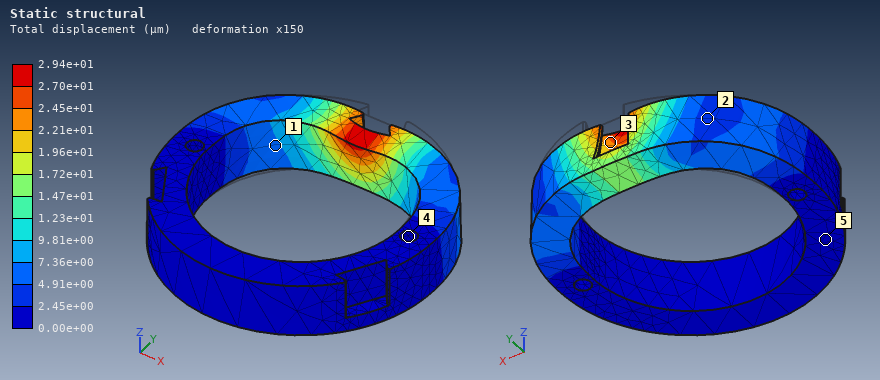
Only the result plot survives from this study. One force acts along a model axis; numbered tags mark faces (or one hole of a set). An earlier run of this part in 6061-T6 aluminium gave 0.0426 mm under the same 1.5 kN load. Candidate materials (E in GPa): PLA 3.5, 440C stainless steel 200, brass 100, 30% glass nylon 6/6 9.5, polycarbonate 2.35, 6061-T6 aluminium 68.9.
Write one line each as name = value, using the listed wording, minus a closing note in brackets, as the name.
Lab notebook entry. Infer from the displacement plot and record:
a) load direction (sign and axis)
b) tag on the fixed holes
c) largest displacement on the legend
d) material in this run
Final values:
load direction = -Y
tag on the fixed holes = 4
largest displacement on the legend = 2.94e+01 µm
material in this run = brass
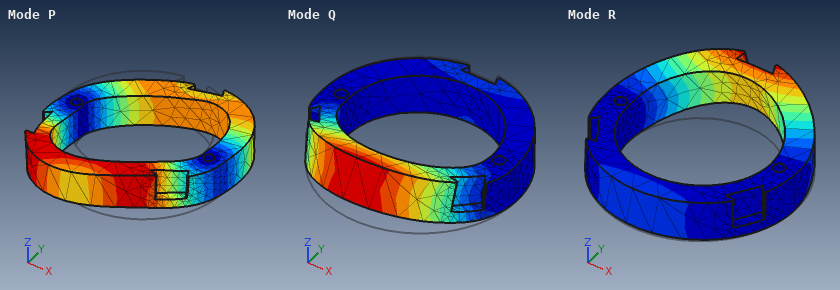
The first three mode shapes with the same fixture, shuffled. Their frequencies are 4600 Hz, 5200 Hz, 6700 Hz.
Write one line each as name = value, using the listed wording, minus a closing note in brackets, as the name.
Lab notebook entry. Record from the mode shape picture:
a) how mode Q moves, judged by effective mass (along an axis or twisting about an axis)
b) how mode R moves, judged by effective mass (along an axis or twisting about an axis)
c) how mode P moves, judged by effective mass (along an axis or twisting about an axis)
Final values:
how mode Q moves, judged by effective mass = along Z
how mode R moves, judged by effective mass = along Z
how mode P moves, judged by effective mass = twisting about Z
